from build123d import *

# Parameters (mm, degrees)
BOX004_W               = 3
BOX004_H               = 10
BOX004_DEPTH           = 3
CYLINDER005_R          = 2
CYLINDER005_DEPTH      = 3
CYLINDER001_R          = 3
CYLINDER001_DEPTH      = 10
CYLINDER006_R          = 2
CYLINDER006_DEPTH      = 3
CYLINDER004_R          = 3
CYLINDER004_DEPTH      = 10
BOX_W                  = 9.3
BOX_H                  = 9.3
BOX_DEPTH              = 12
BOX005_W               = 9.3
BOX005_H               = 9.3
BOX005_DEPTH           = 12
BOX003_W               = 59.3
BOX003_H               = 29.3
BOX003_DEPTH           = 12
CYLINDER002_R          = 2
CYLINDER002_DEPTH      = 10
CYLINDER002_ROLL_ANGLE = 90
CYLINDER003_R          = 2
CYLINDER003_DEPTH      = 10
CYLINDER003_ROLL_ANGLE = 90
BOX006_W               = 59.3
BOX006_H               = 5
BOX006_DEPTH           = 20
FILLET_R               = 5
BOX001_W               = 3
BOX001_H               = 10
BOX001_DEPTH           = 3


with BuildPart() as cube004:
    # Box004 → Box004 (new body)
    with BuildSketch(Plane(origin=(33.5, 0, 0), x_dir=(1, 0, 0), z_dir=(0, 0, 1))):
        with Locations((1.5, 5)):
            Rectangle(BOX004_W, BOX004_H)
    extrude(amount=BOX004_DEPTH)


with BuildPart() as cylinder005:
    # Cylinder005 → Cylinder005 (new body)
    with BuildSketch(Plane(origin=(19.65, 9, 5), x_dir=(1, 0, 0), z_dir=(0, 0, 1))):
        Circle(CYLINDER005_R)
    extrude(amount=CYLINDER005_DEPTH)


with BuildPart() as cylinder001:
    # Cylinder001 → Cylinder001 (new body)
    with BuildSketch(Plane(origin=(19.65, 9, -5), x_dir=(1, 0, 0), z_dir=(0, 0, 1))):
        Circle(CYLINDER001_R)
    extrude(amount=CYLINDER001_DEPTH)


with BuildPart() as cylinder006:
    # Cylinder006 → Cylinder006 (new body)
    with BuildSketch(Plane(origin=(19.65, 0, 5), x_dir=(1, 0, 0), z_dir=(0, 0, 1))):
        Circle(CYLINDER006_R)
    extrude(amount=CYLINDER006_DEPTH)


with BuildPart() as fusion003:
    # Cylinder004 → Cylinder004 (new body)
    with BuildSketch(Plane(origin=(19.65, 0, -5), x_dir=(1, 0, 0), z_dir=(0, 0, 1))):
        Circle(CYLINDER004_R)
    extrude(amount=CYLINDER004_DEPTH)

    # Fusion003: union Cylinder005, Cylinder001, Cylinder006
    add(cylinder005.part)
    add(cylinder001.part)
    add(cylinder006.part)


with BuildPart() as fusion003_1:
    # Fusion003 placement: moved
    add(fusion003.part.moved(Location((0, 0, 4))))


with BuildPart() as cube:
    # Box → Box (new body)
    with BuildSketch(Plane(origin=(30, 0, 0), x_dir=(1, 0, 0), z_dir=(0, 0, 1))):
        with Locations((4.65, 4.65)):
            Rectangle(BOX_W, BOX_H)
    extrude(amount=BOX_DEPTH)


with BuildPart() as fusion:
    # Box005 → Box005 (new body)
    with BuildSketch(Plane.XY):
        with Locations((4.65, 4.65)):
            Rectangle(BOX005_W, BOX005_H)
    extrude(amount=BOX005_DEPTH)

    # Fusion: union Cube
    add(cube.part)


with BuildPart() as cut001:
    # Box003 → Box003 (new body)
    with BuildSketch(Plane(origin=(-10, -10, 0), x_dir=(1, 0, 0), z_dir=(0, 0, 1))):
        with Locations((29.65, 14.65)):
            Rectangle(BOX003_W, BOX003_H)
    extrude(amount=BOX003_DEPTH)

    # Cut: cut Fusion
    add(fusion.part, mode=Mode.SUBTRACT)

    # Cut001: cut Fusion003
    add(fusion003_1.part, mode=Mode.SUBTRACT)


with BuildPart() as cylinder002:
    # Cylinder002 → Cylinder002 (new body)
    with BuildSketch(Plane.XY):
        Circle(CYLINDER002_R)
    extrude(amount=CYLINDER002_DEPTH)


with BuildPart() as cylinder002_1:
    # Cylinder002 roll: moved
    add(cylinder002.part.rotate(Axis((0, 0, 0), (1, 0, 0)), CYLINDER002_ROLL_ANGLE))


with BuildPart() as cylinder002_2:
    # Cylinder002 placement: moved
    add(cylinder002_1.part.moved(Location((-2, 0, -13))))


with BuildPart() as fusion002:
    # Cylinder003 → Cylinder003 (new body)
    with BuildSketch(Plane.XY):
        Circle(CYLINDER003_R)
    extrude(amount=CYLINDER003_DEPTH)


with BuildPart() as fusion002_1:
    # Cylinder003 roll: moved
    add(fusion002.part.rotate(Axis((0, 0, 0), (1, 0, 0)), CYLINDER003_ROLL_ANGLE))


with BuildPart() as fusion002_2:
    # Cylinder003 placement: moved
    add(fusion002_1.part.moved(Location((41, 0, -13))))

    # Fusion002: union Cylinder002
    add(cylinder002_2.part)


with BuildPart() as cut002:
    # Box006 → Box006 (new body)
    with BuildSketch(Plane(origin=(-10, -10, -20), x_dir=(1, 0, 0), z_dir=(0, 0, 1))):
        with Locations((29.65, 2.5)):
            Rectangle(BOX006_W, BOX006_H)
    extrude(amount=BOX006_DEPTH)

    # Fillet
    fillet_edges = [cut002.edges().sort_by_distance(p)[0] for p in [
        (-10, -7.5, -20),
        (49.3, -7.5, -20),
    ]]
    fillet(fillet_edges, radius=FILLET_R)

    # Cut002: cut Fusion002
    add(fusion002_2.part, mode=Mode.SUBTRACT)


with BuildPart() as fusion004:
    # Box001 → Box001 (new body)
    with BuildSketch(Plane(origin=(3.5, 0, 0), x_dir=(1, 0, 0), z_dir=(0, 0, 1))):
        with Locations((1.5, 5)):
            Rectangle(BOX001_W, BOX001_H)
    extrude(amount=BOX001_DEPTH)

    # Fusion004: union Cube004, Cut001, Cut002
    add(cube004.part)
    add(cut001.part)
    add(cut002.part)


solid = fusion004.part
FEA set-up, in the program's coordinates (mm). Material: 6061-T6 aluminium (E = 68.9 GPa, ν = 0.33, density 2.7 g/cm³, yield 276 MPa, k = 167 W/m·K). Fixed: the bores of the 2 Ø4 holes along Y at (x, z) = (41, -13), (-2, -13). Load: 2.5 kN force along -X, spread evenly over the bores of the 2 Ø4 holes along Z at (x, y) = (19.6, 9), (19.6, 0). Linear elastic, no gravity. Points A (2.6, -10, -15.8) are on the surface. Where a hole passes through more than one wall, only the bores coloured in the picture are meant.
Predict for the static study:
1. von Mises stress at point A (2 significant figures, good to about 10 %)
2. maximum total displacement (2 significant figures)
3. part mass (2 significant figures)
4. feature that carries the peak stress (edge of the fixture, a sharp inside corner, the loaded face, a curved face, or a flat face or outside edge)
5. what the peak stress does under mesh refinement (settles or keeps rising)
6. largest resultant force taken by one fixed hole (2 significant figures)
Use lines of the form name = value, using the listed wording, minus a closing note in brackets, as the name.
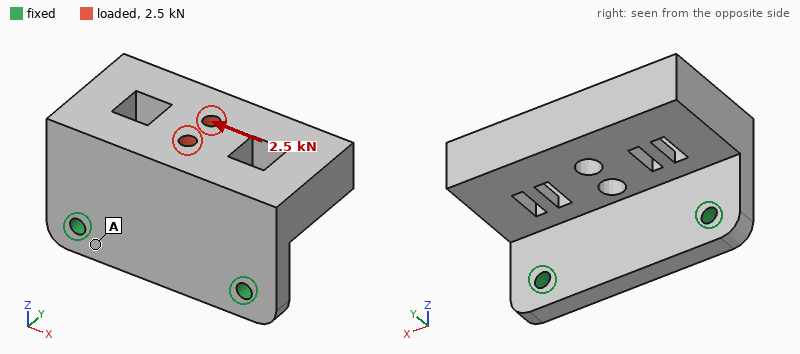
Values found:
von Mises stress at point A = 14 MPa
maximum total displacement = 51 µm
part mass = 65 g
feature that carries the peak stress = edge of the fixture
what the peak stress does under mesh refinement = keeps rising
largest resultant force taken by one fixed hole = 1.9 kN
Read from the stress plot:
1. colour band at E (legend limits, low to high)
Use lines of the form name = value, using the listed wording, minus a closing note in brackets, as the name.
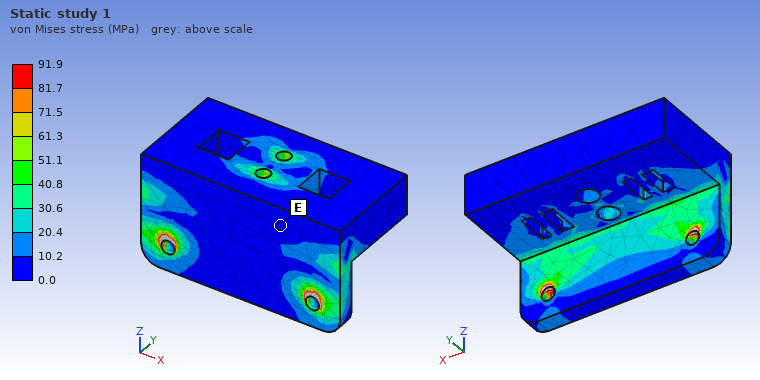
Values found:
colour band at E = 0.0 to 10.2 MPa
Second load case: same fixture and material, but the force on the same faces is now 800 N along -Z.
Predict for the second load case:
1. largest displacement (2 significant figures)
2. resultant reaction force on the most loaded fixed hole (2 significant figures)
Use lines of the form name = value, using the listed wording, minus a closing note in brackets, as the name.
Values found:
largest displacement = 0.14 mm
resultant reaction force on the most loaded fixed hole = 440 N
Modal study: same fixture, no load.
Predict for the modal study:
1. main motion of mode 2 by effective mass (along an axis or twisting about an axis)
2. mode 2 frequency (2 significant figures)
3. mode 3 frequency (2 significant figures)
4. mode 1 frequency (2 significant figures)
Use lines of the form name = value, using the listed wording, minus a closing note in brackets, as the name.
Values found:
main motion of mode 2 by effective mass = along X
mode 2 frequency = 4500 Hz
mode 3 frequency = 7100 Hz
mode 1 frequency = 1700 Hz
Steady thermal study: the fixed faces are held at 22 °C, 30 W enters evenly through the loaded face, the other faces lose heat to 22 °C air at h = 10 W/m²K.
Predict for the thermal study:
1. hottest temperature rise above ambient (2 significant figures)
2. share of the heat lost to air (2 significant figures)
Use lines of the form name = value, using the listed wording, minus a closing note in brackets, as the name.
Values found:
hottest temperature rise above ambient = 25 K
share of the heat lost to air = 3.8 %
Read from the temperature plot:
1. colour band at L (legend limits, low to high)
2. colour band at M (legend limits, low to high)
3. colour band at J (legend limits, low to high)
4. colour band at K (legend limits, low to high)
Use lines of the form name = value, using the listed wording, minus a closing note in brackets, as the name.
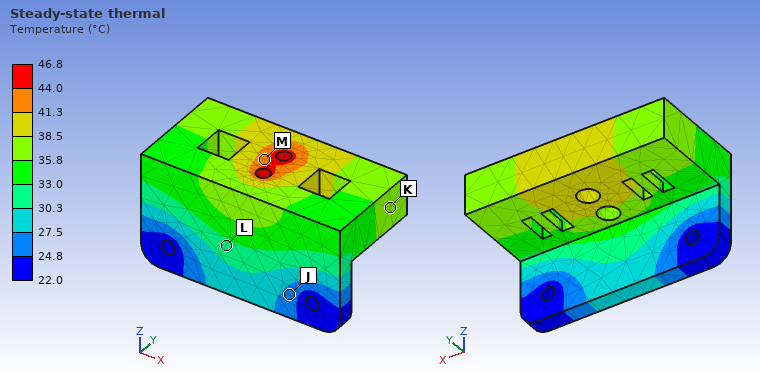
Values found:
colour band at L = 30.3 to 33.0 °C
colour band at M = 41.3 to 44.0 °C
colour band at J = 24.8 to 27.5 °C
colour band at K = 35.8 to 38.5 °C
